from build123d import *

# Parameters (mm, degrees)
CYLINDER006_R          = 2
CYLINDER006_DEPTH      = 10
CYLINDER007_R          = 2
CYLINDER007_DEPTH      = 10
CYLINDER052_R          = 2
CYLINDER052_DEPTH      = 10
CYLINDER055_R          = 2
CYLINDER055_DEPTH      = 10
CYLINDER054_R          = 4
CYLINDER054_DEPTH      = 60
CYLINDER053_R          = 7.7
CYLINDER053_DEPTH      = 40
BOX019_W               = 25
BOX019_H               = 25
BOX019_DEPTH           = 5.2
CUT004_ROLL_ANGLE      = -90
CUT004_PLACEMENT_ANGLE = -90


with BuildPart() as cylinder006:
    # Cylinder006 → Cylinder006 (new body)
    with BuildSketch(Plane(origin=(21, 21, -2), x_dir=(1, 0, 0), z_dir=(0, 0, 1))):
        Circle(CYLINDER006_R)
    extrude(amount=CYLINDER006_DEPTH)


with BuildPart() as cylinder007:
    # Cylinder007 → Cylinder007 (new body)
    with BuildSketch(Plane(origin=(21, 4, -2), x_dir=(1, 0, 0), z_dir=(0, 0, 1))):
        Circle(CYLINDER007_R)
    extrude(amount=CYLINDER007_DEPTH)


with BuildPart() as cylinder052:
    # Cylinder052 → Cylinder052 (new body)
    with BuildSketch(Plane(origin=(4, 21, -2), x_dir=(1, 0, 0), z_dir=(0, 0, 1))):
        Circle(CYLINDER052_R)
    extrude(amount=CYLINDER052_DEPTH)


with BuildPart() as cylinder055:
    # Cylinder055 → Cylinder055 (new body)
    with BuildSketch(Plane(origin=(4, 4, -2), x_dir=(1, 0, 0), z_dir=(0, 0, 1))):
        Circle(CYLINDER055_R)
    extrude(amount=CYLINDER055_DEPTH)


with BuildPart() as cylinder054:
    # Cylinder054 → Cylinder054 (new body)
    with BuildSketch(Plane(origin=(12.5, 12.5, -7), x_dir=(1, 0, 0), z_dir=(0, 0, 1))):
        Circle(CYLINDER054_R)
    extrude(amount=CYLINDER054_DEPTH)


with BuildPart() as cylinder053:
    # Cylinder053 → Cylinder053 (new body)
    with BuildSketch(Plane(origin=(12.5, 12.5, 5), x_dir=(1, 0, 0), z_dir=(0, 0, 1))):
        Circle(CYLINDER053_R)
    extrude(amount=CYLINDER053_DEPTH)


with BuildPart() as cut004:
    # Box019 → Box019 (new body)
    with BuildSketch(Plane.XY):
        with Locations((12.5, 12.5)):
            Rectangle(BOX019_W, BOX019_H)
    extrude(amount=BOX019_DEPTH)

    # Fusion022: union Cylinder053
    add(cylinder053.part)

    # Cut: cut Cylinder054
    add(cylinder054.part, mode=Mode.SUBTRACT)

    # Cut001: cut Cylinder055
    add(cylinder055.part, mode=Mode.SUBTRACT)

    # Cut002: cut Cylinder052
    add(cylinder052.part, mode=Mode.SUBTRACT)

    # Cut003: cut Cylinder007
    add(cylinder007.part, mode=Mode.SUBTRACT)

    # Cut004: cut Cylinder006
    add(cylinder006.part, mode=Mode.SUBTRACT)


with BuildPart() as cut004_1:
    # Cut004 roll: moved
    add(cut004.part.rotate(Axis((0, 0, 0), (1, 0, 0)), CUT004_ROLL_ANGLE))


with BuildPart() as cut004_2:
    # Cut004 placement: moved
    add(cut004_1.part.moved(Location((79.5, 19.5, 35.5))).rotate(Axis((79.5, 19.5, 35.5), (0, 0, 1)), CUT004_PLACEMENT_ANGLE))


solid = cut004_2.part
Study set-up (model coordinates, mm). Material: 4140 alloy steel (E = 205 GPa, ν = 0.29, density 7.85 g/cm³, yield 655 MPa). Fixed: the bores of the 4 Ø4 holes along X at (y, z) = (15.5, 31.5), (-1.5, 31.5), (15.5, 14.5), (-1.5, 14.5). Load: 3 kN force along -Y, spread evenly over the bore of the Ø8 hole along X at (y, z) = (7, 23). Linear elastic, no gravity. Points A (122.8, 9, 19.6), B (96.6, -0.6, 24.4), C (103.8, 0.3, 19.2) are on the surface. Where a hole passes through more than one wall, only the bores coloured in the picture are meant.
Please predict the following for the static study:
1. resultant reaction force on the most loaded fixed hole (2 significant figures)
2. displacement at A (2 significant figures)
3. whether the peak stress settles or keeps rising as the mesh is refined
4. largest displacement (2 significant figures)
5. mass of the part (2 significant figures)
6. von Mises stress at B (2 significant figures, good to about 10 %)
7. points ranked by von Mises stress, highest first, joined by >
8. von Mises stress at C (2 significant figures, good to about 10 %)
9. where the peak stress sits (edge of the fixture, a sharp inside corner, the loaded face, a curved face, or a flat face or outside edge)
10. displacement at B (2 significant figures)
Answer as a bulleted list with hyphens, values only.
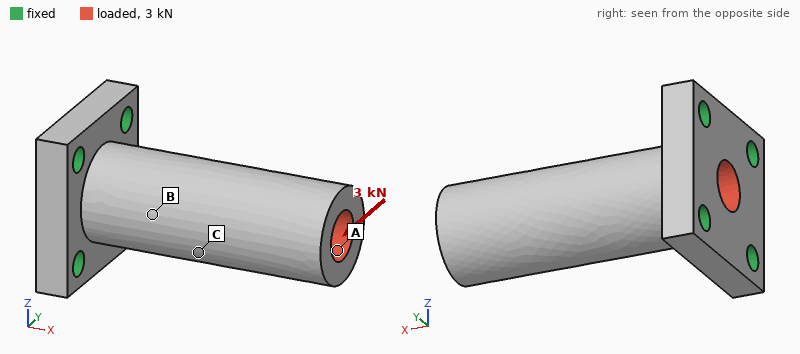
- 2.2 kN
- 72 µm
- keeps rising
- 77 µm
- 64 g
- 75 MPa
- B > C > A
- 39 MPa
- edge of the fixture
- 22 µm
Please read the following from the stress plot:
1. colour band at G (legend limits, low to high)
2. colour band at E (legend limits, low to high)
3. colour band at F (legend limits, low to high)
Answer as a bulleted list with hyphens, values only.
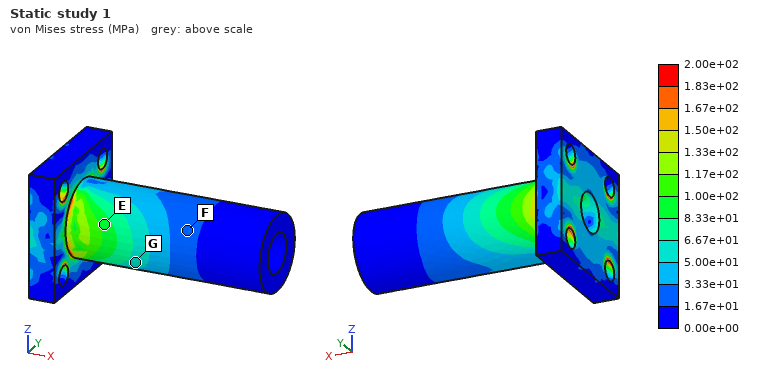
- 5.00e+01 to 6.67e+01 MPa
- 8.33e+01 to 1.00e+02 MPa
- 1.67e+01 to 3.33e+01 MPa
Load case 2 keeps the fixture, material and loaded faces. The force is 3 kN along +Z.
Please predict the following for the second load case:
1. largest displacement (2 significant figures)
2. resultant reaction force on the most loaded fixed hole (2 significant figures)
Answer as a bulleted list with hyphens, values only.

- 77 µm
- 2.2 kN
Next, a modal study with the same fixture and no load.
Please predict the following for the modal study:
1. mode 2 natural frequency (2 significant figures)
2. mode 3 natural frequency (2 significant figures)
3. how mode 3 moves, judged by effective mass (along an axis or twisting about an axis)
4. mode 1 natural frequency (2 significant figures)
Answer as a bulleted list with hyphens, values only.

- 5500 Hz
- 19 kHz
- twisting about X
- 5500 Hz
